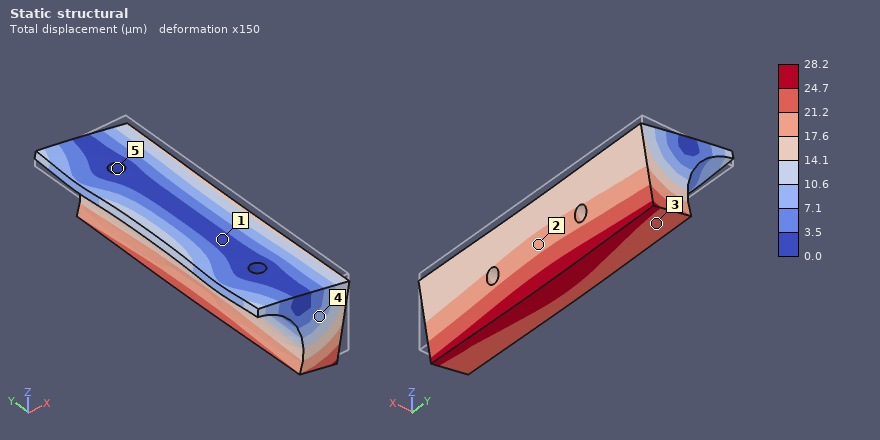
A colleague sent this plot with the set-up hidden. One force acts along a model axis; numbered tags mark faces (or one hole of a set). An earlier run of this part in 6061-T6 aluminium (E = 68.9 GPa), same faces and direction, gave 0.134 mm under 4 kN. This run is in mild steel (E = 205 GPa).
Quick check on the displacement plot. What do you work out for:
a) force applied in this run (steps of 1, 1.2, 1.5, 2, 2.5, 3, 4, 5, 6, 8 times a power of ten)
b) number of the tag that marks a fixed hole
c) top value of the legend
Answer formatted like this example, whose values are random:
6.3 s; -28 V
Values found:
2.5 kN; 5; 28.2 µm
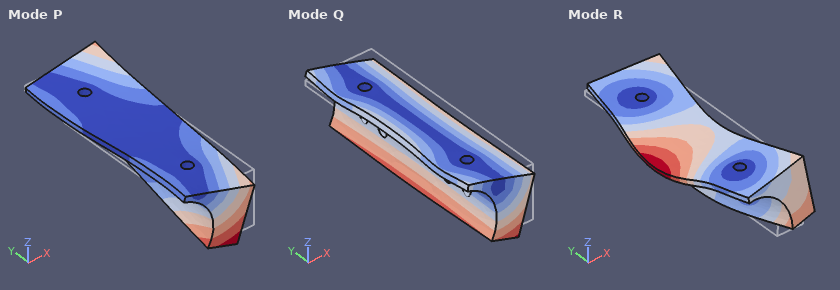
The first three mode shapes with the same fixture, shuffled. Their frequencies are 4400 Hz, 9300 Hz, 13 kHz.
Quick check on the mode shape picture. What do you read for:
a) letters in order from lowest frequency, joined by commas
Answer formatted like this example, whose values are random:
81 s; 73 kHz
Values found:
Q, P, R
